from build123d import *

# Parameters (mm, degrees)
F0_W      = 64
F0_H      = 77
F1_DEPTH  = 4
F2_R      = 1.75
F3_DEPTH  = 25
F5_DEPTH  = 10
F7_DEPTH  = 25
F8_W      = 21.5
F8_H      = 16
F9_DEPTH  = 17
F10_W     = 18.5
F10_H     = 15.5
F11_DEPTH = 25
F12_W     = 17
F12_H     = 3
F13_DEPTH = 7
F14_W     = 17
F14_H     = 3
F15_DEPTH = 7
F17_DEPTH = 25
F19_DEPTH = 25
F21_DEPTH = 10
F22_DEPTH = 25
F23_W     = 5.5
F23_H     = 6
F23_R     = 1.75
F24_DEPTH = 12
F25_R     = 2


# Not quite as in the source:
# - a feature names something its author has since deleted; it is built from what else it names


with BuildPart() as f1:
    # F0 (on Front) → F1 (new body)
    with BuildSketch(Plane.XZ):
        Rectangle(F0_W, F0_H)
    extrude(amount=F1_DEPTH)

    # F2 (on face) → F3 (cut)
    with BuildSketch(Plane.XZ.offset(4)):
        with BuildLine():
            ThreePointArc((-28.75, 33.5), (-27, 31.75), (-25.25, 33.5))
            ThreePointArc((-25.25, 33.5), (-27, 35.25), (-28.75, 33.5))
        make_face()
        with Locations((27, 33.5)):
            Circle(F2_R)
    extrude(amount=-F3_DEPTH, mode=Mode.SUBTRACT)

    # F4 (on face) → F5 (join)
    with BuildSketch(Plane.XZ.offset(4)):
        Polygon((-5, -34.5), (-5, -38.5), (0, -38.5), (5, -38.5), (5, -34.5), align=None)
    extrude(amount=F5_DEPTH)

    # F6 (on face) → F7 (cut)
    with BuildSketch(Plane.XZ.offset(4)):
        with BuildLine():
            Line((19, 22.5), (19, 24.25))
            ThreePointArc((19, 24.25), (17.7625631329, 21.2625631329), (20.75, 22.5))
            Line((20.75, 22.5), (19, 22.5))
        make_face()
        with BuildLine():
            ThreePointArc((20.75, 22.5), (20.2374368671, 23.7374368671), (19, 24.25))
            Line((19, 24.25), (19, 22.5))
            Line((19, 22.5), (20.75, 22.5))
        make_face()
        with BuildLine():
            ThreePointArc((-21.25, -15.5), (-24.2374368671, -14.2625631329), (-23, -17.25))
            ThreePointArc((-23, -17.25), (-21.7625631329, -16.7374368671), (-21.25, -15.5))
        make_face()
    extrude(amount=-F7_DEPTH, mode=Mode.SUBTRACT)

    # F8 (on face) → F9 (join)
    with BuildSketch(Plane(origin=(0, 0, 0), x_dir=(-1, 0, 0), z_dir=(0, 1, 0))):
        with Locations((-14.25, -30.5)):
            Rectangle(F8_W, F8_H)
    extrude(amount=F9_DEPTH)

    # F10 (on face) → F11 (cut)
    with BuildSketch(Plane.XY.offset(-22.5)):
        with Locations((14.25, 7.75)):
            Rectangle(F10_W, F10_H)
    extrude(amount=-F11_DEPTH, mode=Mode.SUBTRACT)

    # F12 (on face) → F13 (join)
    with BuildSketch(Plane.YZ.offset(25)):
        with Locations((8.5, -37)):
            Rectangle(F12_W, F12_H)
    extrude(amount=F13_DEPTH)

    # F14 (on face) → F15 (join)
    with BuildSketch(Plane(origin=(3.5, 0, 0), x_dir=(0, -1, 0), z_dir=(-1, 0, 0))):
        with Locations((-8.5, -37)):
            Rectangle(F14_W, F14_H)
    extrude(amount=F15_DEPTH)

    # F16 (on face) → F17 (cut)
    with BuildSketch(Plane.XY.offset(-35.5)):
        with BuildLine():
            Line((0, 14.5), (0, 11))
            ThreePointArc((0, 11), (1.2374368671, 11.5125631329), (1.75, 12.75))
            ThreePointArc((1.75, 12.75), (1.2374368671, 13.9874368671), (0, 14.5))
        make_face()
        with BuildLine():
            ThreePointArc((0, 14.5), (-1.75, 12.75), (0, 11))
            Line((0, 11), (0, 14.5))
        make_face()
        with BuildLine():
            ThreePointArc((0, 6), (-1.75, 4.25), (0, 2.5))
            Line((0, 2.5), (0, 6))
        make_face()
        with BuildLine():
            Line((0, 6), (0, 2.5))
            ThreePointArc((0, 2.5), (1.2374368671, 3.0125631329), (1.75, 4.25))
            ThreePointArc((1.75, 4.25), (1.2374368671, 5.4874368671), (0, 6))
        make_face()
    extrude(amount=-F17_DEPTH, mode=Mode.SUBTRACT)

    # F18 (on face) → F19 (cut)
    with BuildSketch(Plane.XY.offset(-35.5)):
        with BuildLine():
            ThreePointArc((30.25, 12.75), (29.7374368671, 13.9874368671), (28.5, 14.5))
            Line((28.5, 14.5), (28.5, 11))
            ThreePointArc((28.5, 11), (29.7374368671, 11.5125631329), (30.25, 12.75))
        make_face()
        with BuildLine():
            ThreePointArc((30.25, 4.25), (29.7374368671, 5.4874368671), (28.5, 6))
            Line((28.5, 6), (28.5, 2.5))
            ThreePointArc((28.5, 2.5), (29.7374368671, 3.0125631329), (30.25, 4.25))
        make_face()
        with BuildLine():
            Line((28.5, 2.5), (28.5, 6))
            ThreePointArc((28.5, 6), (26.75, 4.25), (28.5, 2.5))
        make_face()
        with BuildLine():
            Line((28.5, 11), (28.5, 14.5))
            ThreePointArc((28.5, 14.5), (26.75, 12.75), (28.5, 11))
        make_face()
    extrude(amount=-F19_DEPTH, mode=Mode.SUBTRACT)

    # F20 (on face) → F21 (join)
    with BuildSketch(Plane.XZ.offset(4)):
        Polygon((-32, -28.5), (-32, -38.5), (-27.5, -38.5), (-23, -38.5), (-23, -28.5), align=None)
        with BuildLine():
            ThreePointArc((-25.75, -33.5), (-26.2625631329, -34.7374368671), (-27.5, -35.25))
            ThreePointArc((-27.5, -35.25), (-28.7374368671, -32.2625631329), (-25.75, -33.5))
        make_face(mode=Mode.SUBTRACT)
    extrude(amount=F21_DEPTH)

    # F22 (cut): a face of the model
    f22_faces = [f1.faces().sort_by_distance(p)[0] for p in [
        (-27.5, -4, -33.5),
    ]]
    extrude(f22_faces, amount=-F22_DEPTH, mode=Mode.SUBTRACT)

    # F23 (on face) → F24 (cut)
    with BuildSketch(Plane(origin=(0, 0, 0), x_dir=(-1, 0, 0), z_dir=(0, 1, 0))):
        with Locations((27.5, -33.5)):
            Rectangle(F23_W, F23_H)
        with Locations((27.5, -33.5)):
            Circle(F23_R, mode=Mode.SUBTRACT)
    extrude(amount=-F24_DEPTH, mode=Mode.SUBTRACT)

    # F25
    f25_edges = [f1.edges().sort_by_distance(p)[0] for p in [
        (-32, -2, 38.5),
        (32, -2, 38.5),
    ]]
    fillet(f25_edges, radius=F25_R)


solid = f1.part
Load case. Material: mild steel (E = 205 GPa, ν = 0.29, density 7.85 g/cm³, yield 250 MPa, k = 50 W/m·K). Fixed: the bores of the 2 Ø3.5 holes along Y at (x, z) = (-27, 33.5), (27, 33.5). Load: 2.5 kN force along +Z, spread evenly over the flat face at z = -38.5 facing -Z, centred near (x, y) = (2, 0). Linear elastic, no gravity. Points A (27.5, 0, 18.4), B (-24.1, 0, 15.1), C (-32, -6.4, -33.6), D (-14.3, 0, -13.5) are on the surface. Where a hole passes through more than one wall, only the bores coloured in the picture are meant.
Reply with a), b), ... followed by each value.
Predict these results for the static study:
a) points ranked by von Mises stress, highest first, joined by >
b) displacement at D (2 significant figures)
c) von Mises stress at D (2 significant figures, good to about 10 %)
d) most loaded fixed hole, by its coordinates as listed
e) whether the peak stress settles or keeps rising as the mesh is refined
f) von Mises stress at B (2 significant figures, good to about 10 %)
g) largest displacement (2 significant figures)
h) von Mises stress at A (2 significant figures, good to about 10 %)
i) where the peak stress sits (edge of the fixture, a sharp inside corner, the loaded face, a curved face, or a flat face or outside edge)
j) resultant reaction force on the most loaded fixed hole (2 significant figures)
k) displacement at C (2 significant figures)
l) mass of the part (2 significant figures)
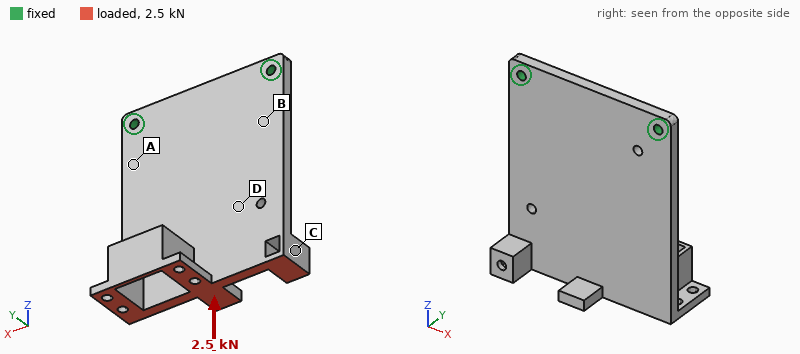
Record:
a) A > B > D > C
b) 0.13 mm
c) 36 MPa
d) (27, 33.5)
e) keeps rising
f) 49 MPa
g) 0.37 mm
h) 66 MPa
i) edge of the fixture
j) 1.4 kN
k) 0.20 mm
l) 180 g
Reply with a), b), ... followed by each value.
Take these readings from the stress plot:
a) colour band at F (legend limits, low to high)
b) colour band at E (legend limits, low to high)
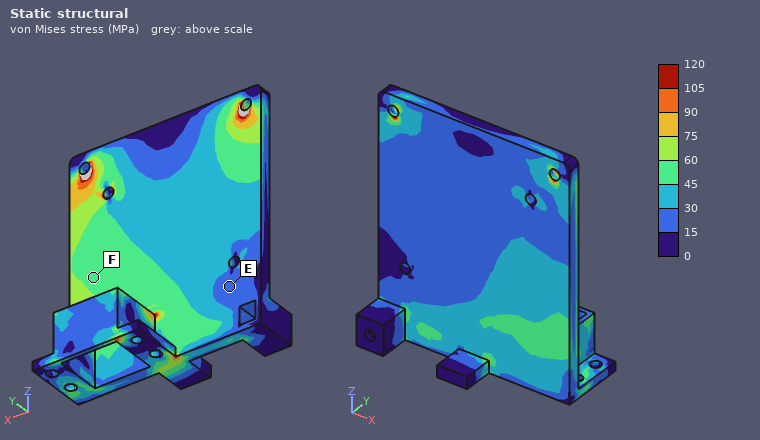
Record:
a) 45 to 60 MPa
b) 15 to 30 MPa
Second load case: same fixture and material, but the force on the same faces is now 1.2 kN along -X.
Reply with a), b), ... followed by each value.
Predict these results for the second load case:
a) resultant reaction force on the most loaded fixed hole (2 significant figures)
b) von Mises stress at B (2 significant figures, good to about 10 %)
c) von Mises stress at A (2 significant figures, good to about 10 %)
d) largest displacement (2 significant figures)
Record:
a) 1.7 kN
b) 20 MPa
c) 25 MPa
d) 80 µm
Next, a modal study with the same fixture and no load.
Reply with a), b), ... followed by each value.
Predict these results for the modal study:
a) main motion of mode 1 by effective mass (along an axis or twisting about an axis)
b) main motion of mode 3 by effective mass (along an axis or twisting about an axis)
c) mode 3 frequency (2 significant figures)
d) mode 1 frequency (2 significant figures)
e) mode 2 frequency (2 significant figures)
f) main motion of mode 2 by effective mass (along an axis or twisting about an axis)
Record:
a) along Y
b) along Y
c) 2800 Hz
d) 440 Hz
e) 1400 Hz
f) twisting about Z
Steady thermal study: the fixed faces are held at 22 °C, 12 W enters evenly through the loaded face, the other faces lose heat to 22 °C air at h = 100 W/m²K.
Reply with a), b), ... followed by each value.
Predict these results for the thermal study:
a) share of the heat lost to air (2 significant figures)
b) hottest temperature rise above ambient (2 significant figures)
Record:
a) 92 %
b) 22 K
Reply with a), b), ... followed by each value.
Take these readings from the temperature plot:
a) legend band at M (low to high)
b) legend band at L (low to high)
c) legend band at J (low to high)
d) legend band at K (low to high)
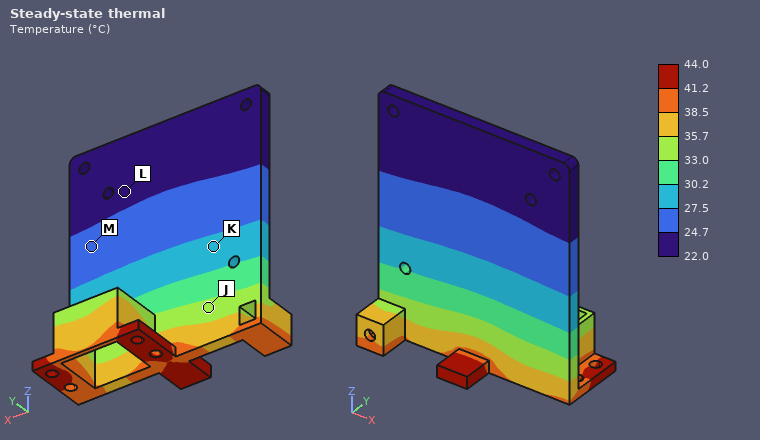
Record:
a) 24.7 to 27.5 °C
b) 22.0 to 24.7 °C
c) 33.0 to 35.7 °C
d) 27.5 to 30.2 °C
